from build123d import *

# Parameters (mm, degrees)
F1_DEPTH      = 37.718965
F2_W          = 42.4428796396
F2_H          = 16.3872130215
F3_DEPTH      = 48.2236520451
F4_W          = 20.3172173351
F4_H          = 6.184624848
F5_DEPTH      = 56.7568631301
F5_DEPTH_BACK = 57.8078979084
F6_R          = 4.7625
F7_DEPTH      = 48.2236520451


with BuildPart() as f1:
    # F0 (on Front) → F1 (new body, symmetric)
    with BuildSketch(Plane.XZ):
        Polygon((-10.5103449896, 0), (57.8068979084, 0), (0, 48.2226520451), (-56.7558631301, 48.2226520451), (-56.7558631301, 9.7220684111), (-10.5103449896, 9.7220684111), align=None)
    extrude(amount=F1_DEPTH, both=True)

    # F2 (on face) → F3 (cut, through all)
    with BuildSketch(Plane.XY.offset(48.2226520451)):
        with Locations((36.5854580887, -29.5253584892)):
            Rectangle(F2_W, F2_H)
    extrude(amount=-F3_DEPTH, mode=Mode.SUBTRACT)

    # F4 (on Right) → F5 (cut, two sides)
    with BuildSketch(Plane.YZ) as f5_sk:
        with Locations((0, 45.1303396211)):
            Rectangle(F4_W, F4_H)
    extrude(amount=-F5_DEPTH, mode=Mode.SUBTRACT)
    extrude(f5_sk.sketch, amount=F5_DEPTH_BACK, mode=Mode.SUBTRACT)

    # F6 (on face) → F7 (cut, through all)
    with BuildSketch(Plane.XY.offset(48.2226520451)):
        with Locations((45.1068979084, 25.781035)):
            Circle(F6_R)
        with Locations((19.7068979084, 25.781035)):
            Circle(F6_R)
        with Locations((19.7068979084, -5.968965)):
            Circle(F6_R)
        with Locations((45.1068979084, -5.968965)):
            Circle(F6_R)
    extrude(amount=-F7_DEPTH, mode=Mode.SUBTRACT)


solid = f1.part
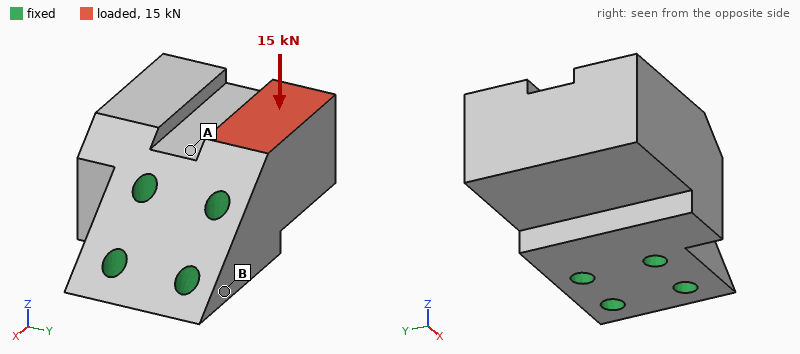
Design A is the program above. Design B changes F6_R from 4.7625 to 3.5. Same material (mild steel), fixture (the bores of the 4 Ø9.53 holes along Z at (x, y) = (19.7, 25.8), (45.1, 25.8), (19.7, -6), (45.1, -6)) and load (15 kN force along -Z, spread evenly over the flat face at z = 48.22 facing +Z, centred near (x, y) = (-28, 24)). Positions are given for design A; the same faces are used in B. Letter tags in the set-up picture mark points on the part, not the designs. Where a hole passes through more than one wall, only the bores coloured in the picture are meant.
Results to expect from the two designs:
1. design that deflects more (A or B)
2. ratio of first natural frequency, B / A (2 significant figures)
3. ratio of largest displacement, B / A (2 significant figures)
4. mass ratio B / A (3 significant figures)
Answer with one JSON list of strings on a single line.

["B", "0.92", "1.1", "1.01"]
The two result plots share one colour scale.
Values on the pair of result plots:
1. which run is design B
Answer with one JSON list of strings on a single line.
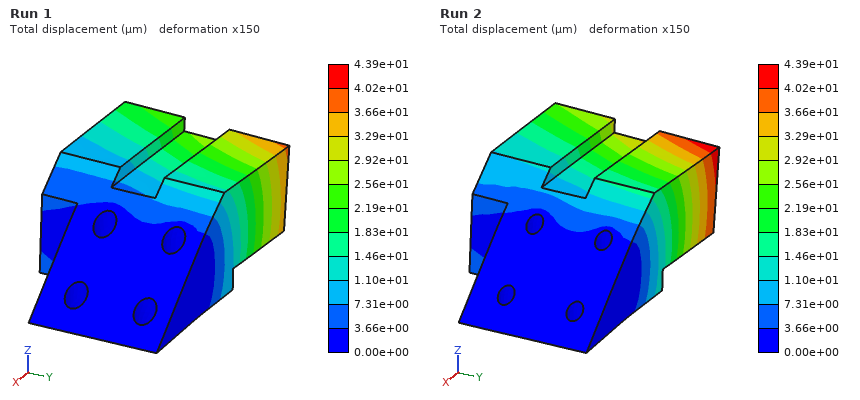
["Run 2"]
